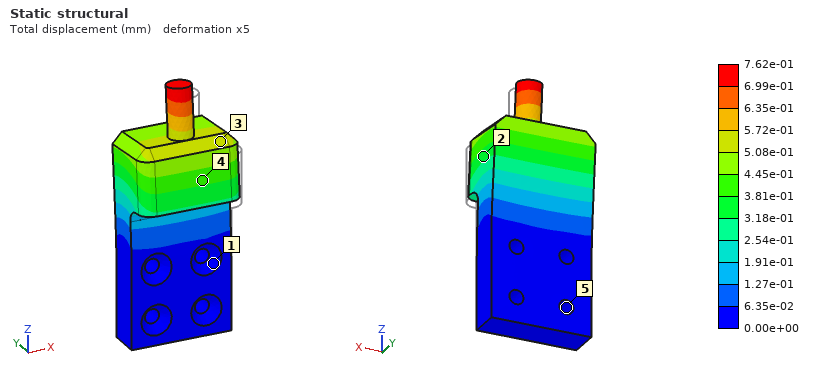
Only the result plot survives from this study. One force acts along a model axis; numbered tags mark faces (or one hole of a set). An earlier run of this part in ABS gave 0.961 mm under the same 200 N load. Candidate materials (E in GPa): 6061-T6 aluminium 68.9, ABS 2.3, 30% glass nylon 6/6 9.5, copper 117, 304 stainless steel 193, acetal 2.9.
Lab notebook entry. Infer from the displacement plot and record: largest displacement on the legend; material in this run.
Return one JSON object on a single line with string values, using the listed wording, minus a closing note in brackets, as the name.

{"largest displacement on the legend": "7.62e-01 mm", "material in this run": "acetal"}
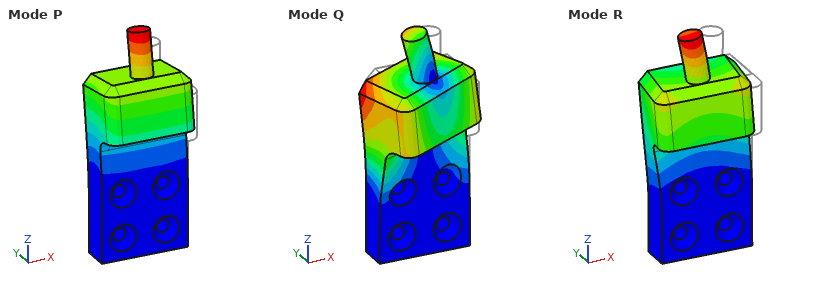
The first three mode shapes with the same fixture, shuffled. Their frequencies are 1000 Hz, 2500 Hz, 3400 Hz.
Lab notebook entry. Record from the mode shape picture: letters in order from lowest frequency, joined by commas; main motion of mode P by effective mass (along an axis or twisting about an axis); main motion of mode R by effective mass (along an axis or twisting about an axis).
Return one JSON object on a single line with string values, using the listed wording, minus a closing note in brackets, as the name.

{"letters in order from lowest frequency, joined by commas": "P, R, Q", "main motion of mode P by effective mass": "along Y", "main motion of mode R by effective mass": "along X"}
